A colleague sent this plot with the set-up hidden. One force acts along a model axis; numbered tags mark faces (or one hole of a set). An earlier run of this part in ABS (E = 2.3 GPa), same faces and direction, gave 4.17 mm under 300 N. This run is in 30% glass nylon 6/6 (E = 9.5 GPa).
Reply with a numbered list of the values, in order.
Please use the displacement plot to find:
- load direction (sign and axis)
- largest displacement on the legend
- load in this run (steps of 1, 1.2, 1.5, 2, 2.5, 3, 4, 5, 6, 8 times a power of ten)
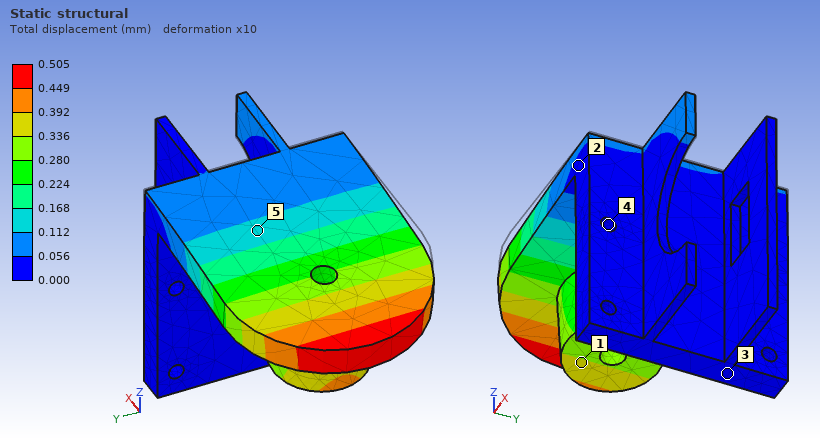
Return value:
1. -Z
2. 0.505 mm
3. 150 N
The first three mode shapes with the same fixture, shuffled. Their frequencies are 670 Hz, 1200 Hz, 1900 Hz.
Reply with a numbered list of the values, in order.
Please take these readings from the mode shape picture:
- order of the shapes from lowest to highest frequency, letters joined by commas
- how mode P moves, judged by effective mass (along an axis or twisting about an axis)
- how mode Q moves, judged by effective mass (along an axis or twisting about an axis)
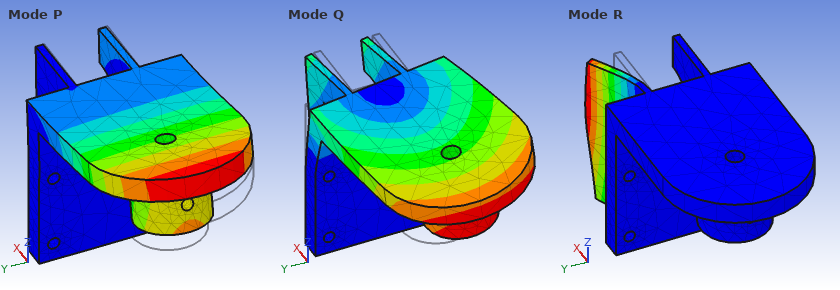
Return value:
1. P, Q, R
2. along Z
3. along Y
